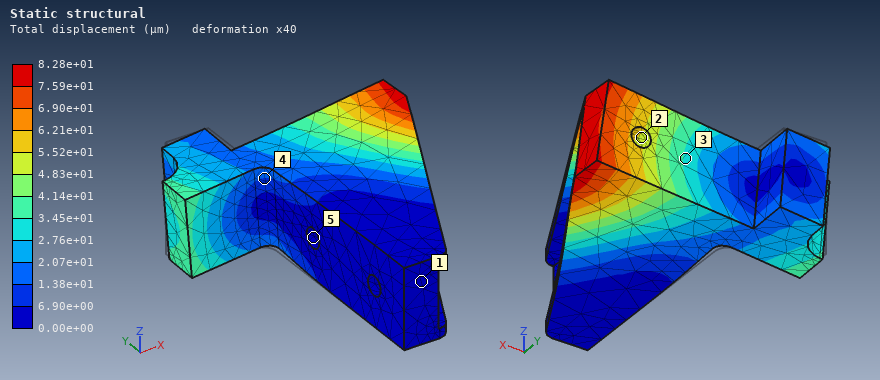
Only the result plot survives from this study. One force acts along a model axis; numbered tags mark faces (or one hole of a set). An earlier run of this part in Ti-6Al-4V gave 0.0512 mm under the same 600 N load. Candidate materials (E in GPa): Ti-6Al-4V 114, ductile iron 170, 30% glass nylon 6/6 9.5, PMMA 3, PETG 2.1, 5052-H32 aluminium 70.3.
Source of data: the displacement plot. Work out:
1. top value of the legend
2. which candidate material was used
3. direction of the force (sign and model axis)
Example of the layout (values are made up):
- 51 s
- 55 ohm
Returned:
- 8.28e+01 µm
- 5052-H32 aluminium
- +Z
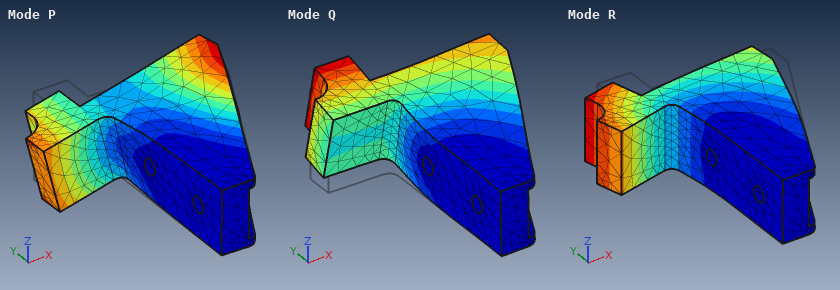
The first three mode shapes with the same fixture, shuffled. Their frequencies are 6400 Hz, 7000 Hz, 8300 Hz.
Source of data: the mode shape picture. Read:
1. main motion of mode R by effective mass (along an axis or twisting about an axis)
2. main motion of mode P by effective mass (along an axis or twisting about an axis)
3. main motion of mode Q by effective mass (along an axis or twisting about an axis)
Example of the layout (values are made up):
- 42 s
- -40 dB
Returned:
- along X
- twisting about Y
- along Z
